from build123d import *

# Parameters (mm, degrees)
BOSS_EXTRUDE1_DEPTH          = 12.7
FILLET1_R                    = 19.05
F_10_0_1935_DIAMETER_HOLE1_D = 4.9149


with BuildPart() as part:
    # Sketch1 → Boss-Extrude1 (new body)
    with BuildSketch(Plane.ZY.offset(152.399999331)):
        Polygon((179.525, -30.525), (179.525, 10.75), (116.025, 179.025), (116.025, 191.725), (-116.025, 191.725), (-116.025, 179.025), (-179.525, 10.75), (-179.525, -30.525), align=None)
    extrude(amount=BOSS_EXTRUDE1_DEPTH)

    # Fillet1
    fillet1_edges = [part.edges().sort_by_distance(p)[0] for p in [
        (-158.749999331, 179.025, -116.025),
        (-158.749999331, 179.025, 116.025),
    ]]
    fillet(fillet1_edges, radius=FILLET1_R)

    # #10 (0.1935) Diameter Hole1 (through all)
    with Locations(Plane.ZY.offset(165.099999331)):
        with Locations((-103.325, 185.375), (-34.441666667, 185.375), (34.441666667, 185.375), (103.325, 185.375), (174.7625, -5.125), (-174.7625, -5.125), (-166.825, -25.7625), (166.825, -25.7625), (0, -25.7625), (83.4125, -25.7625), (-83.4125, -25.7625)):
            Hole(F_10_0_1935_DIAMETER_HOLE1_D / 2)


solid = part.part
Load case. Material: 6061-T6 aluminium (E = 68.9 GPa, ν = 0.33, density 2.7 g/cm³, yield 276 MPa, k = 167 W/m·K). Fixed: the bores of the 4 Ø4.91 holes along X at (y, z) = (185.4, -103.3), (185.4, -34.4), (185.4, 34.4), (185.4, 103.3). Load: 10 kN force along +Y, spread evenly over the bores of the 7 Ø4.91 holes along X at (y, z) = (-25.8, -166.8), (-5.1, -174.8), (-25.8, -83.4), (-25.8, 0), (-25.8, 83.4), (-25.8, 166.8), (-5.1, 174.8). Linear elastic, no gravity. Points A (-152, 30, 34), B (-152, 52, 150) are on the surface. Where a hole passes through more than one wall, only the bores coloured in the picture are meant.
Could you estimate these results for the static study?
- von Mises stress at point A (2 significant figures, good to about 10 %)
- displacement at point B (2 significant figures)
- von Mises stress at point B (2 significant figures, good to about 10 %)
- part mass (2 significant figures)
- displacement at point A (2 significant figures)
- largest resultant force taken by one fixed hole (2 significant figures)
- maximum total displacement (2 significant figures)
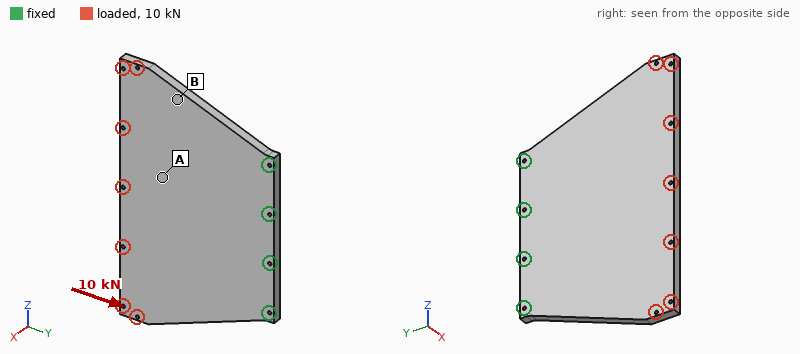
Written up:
1.7 MPa
13 µm
5.7 MPa
2.3 kg
5.8 µm
2.7 kN
26 µm
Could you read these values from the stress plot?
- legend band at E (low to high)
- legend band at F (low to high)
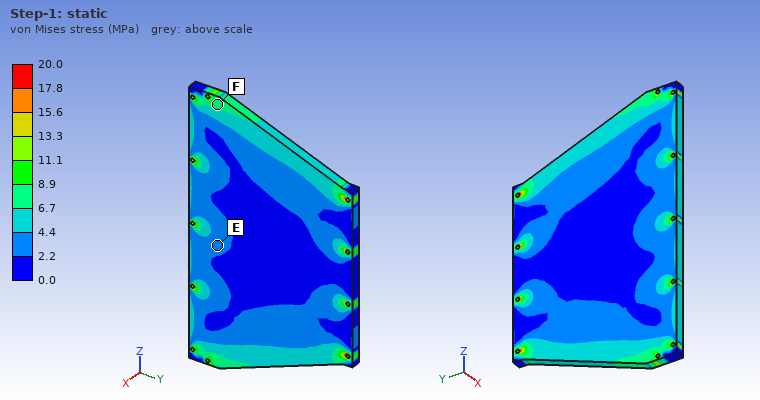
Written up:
2.2 to 4.4 MPa
6.7 to 8.9 MPa
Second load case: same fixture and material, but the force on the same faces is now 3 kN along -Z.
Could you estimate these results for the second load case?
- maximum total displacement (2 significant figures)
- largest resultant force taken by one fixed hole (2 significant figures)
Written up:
29 µm
2.8 kN
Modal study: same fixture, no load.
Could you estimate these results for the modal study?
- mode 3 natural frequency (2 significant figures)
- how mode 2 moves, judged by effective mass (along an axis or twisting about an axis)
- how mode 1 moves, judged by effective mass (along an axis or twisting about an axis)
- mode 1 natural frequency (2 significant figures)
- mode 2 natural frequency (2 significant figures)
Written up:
750 Hz
twisting about Y
along X
170 Hz
300 Hz
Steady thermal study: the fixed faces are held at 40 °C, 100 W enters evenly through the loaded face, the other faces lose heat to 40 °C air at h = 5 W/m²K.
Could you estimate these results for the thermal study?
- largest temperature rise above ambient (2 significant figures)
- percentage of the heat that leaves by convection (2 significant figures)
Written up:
44 K
15 %
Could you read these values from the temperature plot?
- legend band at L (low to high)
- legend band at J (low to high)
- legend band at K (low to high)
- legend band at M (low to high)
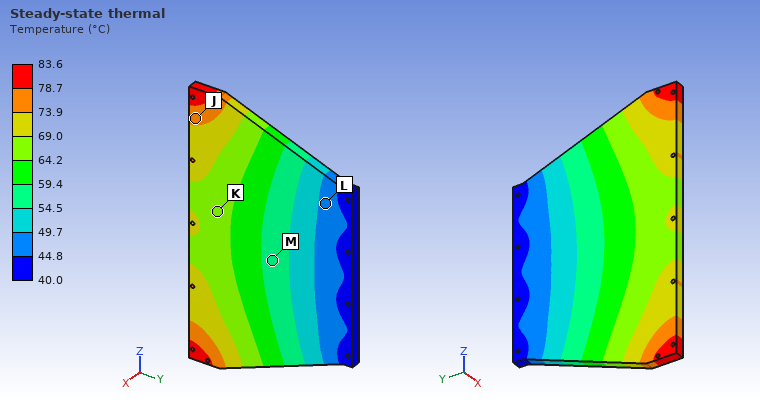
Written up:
44.8 to 49.7 °C
73.9 to 78.7 °C
64.2 to 69.0 °C
54.5 to 59.4 °C
